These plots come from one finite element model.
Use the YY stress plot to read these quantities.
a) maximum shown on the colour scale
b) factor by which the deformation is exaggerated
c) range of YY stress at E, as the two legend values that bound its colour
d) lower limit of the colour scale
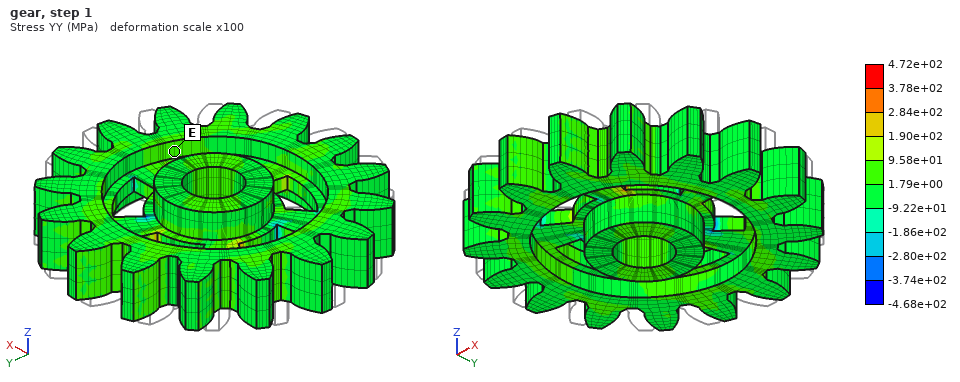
4.72e+02 MPa
100
1.79e+00 to 9.58e+01 MPa
-4.68e+02 MPa
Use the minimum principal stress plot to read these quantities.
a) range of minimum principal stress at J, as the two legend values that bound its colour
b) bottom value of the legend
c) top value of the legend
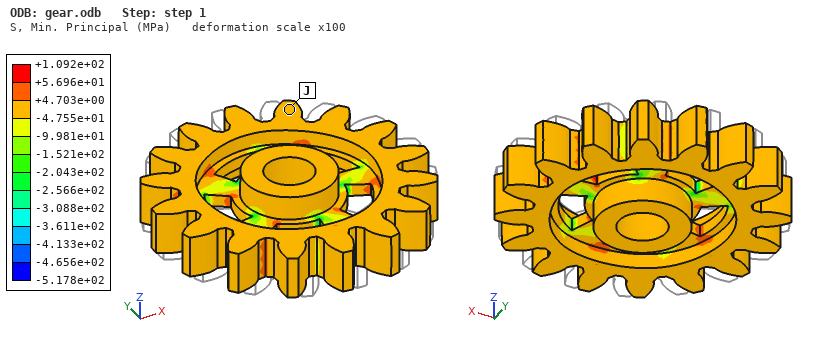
-4.755e+01 to +4.703e+00 MPa
-5.178e+02 MPa
+1.092e+02 MPa
